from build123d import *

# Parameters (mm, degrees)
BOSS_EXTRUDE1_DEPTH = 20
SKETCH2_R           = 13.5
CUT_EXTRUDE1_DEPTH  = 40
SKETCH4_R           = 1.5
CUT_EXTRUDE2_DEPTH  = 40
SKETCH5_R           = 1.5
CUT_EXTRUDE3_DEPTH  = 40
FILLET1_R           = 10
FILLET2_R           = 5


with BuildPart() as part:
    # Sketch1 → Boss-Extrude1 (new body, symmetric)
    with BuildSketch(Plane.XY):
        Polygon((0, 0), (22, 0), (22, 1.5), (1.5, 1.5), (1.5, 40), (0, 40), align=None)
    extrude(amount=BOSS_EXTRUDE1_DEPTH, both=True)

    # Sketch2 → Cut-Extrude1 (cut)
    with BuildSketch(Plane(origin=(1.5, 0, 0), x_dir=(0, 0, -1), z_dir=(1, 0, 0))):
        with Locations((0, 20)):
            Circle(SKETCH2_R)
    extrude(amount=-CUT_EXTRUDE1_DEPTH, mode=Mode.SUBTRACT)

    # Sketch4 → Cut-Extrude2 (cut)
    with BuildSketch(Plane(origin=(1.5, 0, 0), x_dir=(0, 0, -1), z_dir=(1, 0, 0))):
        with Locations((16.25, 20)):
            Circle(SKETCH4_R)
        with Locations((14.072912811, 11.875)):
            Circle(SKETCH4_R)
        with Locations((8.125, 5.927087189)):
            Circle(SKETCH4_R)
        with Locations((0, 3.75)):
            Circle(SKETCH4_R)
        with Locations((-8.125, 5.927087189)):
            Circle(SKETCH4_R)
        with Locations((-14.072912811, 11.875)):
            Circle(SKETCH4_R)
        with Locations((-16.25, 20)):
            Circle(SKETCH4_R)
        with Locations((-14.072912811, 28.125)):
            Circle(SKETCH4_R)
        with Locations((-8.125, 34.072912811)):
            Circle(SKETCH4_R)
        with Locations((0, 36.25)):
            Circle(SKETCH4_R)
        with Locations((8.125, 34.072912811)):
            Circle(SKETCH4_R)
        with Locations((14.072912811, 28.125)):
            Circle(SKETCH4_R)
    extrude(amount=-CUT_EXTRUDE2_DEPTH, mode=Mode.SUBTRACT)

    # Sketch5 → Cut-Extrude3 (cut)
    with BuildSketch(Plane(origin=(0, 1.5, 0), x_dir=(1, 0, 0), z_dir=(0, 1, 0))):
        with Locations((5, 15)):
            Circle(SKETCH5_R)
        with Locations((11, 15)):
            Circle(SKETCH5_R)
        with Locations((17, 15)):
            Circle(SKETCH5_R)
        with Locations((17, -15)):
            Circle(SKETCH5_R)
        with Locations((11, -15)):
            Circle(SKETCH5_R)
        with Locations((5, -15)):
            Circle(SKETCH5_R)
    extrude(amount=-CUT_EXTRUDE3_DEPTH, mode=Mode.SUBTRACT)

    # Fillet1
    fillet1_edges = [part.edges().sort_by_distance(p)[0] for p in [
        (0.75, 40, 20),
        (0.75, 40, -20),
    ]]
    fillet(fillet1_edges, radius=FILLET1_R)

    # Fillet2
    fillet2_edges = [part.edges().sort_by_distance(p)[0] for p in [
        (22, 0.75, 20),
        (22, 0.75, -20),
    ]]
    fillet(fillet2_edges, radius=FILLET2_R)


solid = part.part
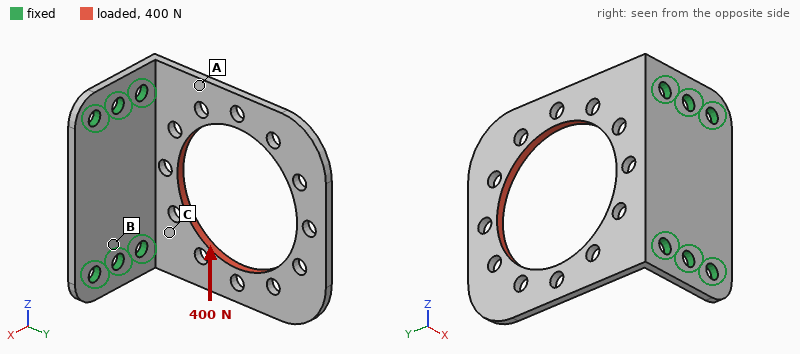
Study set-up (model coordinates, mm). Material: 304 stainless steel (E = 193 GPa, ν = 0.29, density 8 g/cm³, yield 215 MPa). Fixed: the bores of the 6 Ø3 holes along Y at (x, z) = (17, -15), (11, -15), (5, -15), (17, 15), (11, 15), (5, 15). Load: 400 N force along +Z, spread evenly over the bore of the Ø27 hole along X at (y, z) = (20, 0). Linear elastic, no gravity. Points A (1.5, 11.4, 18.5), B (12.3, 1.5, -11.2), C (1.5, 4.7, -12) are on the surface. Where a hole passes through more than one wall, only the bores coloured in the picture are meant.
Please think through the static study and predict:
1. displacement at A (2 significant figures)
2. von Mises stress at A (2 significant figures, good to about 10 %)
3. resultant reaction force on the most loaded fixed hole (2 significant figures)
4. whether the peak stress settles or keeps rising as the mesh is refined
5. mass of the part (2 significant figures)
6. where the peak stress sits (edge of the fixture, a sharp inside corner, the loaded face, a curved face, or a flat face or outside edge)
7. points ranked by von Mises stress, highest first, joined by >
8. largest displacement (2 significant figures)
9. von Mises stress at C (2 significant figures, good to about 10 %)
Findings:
23 µm
47 MPa
290 N
keeps rising
20 g
edge of the fixture
A > C > B
55 µm
28 MPa
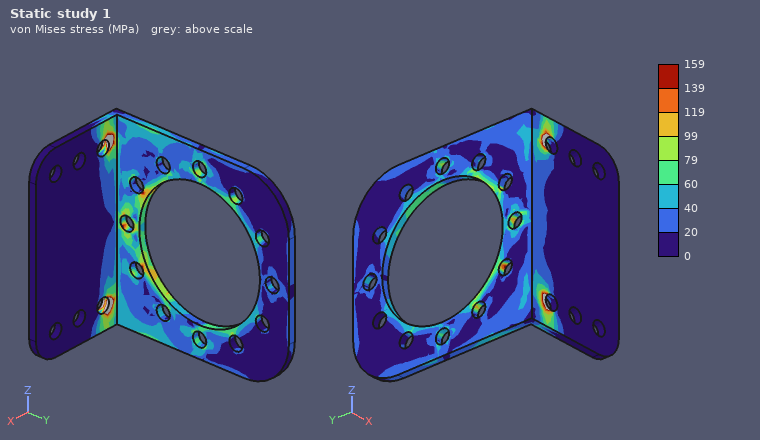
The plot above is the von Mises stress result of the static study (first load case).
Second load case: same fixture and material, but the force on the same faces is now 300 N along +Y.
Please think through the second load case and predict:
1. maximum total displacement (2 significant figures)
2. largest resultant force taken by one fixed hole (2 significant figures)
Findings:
49 µm
170 N
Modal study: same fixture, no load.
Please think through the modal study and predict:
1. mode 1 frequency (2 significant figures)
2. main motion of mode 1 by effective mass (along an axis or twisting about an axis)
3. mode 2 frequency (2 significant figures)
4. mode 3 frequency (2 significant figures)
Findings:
600 Hz
along X
1500 Hz
3700 Hz
